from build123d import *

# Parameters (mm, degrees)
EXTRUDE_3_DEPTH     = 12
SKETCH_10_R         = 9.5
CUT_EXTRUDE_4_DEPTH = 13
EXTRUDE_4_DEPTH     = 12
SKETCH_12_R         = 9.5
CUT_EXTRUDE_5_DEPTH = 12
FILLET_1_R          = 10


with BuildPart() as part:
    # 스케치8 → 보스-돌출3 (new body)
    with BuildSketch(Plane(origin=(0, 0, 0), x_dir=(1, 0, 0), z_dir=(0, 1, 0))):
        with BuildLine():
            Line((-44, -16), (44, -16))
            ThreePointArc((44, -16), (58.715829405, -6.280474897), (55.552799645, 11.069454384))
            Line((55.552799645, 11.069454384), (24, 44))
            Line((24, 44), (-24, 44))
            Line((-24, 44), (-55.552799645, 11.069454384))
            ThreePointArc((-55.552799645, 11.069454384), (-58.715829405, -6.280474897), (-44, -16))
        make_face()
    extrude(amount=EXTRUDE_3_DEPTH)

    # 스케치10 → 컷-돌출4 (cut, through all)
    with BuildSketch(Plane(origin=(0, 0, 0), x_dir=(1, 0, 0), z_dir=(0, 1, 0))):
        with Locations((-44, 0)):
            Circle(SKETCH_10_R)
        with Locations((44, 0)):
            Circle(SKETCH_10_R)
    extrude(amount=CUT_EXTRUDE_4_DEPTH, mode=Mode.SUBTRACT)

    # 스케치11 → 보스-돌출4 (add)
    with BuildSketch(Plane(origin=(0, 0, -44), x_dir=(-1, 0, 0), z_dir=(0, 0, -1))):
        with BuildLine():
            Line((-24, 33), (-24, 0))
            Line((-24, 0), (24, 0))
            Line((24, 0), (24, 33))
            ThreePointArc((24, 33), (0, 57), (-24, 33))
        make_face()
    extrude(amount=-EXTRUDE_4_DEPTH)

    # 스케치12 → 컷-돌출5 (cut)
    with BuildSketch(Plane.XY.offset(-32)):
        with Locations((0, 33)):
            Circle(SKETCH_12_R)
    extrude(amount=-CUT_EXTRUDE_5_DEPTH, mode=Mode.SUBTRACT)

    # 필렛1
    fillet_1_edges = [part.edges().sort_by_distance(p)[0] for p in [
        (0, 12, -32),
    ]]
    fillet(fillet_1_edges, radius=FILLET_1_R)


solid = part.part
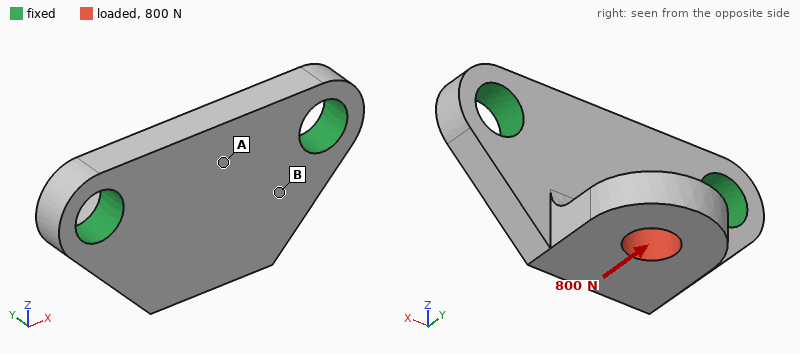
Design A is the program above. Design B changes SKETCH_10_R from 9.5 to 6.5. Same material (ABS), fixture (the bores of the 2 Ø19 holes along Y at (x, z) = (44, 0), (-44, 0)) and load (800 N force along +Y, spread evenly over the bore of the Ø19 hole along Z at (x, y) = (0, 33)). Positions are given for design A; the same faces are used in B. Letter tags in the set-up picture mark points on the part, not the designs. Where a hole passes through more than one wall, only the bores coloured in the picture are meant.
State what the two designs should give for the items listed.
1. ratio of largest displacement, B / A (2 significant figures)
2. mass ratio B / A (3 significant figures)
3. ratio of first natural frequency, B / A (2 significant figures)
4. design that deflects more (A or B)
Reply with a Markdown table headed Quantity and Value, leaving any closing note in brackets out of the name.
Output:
| Quantity | Value |
|---|---|
| ratio of largest displacement, B / A | 1.2 |
| mass ratio B / A | 1.04 |
| ratio of first natural frequency, B / A | 0.91 |
| design that deflects more | B |
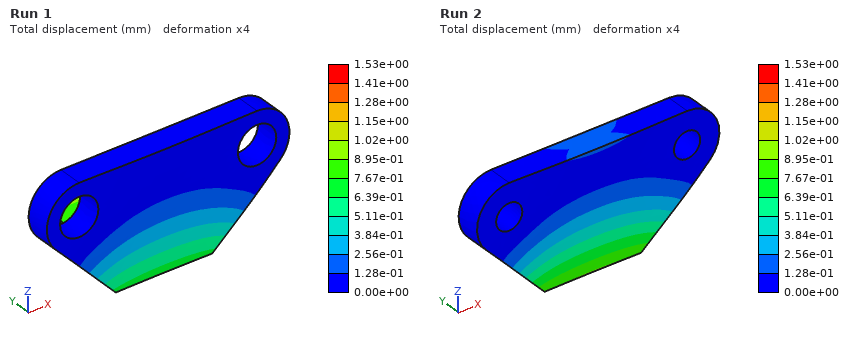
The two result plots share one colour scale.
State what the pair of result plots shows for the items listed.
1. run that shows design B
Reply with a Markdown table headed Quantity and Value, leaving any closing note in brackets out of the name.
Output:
| Quantity | Value |
|---|---|
| run that shows design B | Run 2 |
